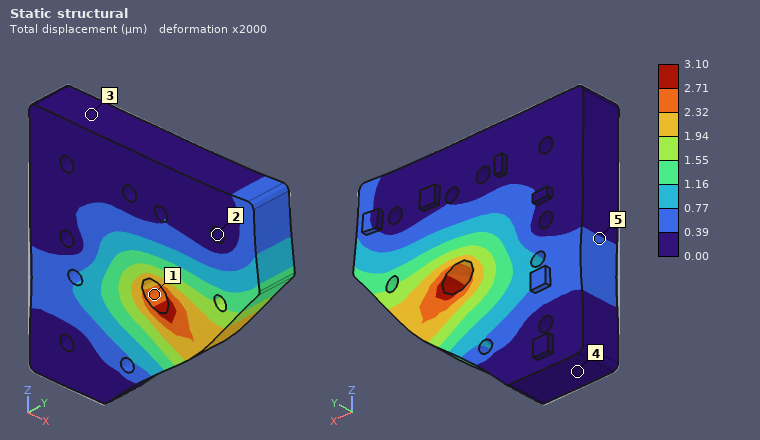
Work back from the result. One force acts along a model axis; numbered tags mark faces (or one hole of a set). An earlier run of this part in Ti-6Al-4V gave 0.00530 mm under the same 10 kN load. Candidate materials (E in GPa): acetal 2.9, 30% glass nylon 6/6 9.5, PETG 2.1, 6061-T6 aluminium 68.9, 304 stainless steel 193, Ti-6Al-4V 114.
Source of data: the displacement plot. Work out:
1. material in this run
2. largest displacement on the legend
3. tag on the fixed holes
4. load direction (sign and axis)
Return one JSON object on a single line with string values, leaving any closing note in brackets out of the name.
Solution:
{"material in this run": "304 stainless steel", "largest displacement on the legend": "3.10 µm", "tag on the fixed holes": "2", "load direction": "+X"}
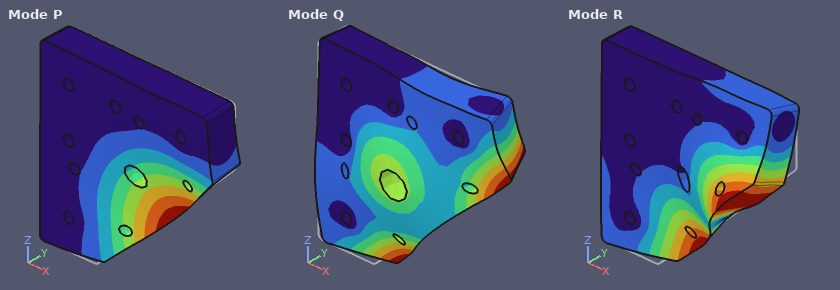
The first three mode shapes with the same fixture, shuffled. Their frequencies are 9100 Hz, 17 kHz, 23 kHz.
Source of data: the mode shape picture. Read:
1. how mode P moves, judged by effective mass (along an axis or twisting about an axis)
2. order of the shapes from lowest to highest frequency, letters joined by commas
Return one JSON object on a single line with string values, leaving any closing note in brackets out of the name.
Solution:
{"how mode P moves, judged by effective mass": "along Y", "order of the shapes from lowest to highest frequency, letters joined by commas": "P, R, Q"}
